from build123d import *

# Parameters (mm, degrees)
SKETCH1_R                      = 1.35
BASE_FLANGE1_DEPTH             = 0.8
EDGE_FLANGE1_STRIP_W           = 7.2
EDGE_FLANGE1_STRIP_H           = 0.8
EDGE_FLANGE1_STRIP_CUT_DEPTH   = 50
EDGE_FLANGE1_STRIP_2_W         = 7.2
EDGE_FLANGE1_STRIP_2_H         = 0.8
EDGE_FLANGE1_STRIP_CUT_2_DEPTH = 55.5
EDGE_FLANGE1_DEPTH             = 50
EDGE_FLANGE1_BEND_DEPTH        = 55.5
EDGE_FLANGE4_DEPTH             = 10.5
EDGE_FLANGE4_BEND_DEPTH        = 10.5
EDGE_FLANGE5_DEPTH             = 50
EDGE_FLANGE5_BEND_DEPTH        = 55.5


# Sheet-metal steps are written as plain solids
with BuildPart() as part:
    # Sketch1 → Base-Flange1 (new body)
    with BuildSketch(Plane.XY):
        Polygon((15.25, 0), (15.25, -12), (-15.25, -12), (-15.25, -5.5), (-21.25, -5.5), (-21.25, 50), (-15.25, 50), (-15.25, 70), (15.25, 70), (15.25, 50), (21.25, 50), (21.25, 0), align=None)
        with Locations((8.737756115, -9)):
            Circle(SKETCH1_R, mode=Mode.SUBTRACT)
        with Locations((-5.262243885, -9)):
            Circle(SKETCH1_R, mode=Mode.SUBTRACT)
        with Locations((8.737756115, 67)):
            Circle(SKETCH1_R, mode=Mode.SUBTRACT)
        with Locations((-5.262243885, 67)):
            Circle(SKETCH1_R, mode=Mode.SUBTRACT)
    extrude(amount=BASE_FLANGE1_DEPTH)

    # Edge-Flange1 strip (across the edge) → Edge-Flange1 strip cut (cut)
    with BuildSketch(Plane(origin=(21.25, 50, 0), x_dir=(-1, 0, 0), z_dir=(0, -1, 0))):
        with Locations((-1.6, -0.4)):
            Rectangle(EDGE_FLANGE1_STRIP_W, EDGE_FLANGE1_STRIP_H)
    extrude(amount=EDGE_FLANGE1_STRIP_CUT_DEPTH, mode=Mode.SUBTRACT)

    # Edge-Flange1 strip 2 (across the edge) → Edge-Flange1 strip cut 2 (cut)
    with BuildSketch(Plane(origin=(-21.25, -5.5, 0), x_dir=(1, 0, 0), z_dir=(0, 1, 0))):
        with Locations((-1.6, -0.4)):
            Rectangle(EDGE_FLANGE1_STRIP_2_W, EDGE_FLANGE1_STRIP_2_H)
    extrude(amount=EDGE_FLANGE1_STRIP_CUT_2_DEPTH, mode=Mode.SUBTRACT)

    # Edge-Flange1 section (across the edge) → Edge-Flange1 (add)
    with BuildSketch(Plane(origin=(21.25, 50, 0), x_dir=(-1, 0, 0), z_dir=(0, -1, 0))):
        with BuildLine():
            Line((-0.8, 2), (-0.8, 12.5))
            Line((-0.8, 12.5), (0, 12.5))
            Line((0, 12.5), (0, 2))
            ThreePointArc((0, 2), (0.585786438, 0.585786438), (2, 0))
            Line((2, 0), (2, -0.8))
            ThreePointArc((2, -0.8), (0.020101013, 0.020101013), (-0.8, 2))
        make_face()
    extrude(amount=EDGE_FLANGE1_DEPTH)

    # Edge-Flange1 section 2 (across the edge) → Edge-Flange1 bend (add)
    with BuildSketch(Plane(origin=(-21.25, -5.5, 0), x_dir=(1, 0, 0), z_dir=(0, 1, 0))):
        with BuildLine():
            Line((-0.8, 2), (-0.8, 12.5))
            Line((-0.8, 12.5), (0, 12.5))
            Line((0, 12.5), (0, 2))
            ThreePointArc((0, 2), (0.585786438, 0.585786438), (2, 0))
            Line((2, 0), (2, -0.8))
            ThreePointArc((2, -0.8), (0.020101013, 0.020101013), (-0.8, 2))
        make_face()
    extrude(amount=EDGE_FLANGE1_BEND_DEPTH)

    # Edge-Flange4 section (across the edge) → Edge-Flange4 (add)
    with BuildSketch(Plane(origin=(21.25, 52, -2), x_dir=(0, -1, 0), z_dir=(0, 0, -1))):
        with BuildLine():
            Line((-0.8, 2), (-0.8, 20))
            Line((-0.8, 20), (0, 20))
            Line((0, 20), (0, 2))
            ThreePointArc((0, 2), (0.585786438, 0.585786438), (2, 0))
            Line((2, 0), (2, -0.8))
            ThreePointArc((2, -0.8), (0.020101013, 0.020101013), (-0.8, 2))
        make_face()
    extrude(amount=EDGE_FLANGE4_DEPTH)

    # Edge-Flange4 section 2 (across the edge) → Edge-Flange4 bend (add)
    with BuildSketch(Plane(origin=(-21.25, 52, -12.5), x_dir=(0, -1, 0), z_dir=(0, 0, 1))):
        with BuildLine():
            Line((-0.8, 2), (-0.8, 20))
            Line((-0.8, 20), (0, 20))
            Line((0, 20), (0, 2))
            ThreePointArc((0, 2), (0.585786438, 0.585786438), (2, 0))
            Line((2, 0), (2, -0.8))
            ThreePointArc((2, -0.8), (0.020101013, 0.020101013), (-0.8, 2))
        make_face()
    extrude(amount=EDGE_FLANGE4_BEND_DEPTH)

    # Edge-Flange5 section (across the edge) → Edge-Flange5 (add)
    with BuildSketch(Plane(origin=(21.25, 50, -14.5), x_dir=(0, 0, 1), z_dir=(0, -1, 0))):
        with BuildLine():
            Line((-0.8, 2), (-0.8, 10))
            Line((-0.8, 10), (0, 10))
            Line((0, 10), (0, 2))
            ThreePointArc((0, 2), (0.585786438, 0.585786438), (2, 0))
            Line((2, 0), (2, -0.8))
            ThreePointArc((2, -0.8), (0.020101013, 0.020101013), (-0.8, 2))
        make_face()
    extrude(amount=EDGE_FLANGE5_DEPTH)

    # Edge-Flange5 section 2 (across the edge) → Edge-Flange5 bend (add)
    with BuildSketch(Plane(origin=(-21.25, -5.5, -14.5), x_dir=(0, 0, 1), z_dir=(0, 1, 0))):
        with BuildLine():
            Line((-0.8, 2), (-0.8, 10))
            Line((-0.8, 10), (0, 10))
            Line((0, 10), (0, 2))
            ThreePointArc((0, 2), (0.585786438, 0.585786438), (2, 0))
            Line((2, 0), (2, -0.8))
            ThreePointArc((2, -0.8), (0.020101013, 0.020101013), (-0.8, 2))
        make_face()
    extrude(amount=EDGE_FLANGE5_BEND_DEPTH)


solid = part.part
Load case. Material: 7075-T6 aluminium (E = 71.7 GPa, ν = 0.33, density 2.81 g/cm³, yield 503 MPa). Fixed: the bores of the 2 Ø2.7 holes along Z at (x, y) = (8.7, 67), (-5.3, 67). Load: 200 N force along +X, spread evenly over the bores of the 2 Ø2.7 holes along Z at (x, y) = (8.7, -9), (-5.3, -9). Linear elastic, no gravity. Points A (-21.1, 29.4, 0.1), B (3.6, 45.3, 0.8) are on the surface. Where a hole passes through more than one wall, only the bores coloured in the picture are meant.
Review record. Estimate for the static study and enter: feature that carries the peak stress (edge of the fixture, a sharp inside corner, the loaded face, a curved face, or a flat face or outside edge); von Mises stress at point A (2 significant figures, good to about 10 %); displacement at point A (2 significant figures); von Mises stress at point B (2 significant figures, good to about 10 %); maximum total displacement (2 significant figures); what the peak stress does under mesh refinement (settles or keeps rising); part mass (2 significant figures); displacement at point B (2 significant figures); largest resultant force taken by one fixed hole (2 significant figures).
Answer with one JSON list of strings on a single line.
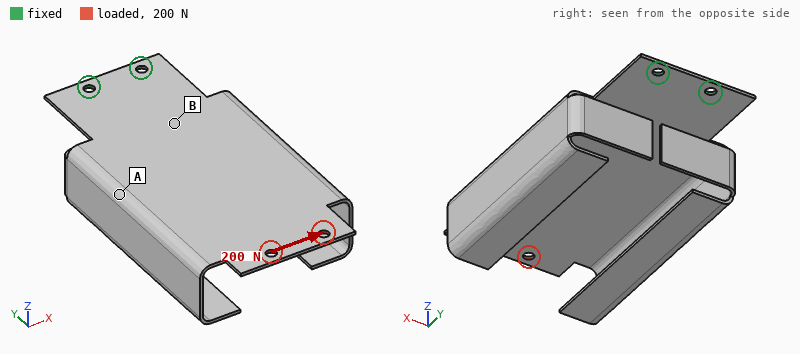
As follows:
["edge of the fixture", "19 MPa", "0.16 mm", "42 MPa", "0.32 mm", "keeps rising", "14 g", "0.065 mm", "960 N"]
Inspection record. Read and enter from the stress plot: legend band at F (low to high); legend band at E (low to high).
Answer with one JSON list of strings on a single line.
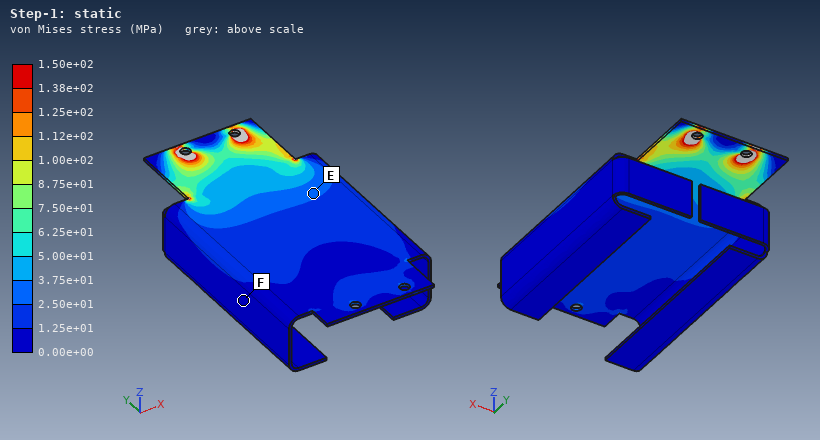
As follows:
["0.00e+00 to 1.25e+01 MPa", "2.50e+01 to 3.75e+01 MPa"]
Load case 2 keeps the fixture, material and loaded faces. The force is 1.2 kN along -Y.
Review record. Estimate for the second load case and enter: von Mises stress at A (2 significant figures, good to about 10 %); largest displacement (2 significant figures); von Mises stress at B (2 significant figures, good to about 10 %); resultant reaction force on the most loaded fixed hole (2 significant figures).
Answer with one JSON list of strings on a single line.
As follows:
["16 MPa", "85 µm", "46 MPa", "600 N"]
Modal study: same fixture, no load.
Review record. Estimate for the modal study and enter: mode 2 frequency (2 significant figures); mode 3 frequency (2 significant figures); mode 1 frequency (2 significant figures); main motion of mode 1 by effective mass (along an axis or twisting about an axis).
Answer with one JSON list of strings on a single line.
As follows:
["210 Hz", "580 Hz", "78 Hz", "along Z"]
